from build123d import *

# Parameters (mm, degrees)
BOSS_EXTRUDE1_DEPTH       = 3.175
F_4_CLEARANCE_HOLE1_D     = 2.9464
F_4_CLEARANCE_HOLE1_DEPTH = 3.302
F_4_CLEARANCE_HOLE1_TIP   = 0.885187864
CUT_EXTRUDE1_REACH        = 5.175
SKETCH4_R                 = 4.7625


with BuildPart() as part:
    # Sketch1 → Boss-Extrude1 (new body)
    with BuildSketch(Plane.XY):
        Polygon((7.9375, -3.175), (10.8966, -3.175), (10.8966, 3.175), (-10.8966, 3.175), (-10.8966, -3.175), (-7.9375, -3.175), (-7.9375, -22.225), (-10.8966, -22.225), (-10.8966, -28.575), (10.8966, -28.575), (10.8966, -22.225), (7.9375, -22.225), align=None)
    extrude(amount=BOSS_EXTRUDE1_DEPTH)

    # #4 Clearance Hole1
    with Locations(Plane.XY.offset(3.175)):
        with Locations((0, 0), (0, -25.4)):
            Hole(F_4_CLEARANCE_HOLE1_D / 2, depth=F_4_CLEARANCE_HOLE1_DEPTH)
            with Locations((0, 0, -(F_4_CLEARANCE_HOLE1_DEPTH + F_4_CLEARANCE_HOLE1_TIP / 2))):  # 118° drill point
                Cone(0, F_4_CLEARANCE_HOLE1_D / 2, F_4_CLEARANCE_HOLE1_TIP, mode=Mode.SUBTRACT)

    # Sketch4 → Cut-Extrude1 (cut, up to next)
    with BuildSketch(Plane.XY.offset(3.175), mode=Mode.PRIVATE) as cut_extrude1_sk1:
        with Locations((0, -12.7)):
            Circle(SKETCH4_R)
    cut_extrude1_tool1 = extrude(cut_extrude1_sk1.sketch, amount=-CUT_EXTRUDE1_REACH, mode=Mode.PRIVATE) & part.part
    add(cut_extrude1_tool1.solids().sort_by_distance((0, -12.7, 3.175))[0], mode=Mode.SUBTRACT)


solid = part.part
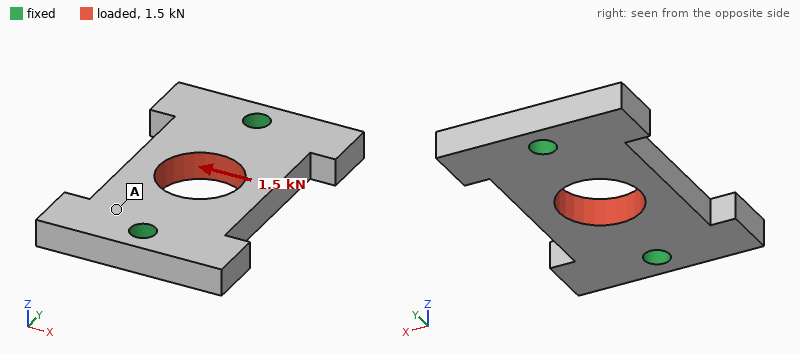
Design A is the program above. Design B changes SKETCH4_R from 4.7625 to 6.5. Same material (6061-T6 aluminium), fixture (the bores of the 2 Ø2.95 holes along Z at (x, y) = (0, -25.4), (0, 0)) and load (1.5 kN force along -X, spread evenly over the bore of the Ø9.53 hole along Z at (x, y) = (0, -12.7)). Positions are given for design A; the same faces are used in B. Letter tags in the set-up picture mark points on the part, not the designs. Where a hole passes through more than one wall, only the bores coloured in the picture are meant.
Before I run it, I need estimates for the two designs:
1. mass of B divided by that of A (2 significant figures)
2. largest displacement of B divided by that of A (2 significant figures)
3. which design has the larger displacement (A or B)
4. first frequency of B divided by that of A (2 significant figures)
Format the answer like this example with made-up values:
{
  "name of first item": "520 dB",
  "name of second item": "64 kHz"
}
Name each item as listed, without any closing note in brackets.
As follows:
{
  "mass of B divided by that of A": "0.88",
  "largest displacement of B divided by that of A": "1.4",
  "which design has the larger displacement": "B",
  "first frequency of B divided by that of A": "1.0"
}
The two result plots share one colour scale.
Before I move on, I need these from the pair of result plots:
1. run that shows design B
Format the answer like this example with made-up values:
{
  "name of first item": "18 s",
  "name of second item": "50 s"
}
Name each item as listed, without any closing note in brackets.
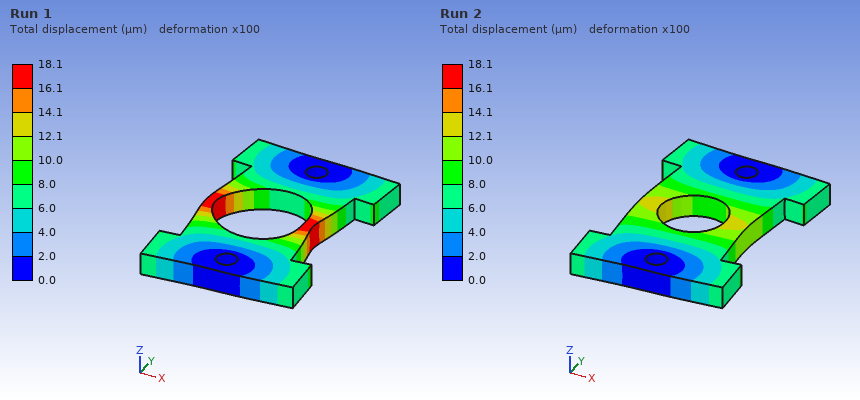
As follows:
{
  "run that shows design B": "Run 1"
}
